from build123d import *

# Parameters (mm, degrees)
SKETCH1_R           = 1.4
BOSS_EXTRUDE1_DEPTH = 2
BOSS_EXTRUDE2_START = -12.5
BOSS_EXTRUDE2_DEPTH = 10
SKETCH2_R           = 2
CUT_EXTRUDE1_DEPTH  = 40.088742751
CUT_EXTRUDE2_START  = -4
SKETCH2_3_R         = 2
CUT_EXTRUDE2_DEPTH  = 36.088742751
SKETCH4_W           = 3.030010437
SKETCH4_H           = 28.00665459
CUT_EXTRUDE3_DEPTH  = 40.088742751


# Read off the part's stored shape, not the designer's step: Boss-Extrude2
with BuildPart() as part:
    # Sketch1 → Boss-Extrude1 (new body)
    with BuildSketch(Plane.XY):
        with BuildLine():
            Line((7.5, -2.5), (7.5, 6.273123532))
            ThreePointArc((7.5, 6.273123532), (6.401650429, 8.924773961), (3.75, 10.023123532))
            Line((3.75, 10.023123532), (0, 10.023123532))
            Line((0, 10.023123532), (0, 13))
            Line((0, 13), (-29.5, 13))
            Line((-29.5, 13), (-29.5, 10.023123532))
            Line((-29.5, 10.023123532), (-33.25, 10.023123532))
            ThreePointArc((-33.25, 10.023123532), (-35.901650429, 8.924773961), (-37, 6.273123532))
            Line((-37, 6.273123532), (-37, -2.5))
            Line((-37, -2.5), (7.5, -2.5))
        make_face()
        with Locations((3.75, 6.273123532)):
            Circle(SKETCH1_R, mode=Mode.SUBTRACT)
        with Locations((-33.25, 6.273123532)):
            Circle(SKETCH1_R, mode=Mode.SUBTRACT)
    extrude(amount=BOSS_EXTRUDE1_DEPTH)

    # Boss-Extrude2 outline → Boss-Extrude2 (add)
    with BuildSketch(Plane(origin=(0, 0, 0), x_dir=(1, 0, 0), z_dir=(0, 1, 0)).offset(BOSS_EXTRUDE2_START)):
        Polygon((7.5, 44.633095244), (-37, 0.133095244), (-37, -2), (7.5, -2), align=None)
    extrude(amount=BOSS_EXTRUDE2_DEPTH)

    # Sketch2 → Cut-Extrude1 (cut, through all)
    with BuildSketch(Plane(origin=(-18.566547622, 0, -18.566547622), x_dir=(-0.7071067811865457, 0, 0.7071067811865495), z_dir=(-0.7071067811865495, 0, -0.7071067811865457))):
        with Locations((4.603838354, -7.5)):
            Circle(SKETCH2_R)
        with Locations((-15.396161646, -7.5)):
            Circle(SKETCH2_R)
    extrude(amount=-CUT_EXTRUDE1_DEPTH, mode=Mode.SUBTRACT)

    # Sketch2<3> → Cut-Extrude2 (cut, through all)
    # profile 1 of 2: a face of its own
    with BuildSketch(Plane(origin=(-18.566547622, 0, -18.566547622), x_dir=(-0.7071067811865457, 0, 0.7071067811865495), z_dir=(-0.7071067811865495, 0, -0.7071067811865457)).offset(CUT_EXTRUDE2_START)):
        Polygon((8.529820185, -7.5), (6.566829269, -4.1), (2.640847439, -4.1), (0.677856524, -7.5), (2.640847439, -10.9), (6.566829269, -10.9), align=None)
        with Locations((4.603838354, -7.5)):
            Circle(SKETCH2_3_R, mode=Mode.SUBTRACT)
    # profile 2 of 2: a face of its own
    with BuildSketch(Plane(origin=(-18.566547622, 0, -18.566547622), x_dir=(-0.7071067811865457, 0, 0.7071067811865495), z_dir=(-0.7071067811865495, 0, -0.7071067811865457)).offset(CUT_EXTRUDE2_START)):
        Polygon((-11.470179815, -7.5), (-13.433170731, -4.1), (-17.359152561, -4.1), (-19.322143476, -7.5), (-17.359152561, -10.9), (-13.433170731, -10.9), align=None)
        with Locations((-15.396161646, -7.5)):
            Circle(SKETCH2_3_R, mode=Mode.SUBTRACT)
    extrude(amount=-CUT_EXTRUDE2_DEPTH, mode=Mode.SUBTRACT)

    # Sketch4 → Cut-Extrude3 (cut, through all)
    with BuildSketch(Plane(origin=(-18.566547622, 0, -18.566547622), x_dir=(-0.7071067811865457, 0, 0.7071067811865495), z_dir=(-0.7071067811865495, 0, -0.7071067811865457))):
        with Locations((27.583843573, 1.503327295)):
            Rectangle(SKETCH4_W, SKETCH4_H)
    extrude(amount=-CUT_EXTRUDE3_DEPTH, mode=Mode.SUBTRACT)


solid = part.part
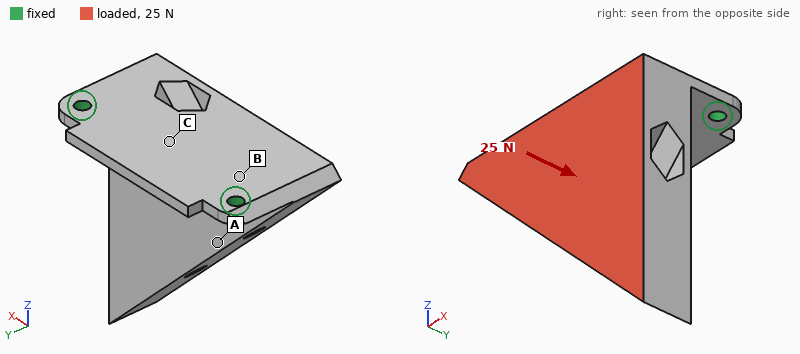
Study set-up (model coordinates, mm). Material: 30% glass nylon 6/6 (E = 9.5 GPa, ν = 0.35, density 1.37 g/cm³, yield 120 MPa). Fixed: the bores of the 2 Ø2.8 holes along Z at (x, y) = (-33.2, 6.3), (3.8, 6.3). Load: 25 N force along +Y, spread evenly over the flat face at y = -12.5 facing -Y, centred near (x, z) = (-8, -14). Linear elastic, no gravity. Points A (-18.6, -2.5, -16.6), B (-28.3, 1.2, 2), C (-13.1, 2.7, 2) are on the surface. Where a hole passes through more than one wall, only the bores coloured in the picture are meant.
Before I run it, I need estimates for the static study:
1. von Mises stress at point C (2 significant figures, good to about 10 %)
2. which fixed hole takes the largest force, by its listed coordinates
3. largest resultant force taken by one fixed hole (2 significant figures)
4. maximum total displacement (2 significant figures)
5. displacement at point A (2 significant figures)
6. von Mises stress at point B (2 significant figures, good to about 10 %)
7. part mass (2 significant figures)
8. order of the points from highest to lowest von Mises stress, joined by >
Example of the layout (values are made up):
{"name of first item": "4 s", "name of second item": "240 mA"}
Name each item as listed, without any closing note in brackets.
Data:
{"von Mises stress at point C": "6.5 MPa", "which fixed hole takes the largest force, by its listed coordinates": "(3.8, 6.3)", "largest resultant force taken by one fixed hole": "18 N", "maximum total displacement": "0.80 mm", "displacement at point A": "0.30 mm", "von Mises stress at point B": "12 MPa", "part mass": "14 g", "order of the points from highest to lowest von Mises stress, joined by >": "B > C > A"}
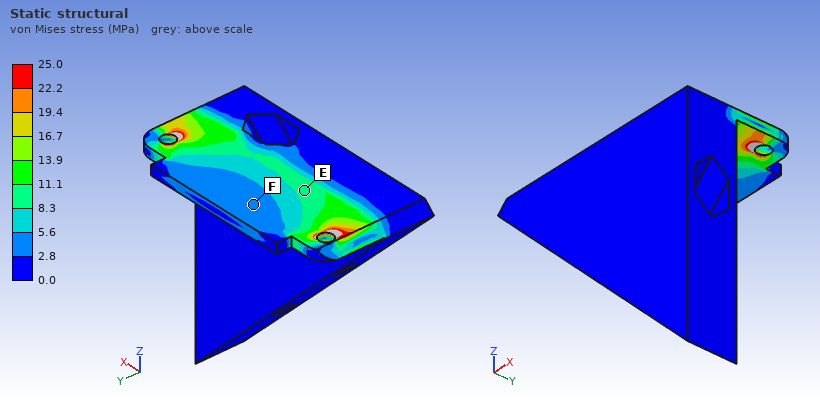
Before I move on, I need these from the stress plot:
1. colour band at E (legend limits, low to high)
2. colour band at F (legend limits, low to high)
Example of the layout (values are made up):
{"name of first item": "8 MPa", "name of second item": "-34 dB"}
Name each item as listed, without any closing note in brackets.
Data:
{"colour band at E": "8.3 to 11.1 MPa", "colour band at F": "2.8 to 5.6 MPa"}
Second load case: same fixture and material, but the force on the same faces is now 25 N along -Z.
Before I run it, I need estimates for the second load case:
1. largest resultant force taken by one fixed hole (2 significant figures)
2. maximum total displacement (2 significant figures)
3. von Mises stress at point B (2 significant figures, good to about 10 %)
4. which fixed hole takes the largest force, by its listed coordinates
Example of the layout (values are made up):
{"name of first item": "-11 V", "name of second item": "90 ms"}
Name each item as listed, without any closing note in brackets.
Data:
{"largest resultant force taken by one fixed hole": "17 N", "maximum total displacement": "0.78 mm", "von Mises stress at point B": "12 MPa", "which fixed hole takes the largest force, by its listed coordinates": "(3.8, 6.3)"}
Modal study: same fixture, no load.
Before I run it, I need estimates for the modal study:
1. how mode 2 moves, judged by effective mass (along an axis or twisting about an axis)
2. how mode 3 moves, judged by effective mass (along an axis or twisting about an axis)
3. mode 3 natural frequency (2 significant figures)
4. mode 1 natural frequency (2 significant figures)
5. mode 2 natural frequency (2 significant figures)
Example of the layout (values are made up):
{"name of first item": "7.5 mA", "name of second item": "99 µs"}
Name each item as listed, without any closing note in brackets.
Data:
{"how mode 2 moves, judged by effective mass": "along X", "how mode 3 moves, judged by effective mass": "along Z", "mode 3 natural frequency": "2000 Hz", "mode 1 natural frequency": "320 Hz", "mode 2 natural frequency": "1400 Hz"}
